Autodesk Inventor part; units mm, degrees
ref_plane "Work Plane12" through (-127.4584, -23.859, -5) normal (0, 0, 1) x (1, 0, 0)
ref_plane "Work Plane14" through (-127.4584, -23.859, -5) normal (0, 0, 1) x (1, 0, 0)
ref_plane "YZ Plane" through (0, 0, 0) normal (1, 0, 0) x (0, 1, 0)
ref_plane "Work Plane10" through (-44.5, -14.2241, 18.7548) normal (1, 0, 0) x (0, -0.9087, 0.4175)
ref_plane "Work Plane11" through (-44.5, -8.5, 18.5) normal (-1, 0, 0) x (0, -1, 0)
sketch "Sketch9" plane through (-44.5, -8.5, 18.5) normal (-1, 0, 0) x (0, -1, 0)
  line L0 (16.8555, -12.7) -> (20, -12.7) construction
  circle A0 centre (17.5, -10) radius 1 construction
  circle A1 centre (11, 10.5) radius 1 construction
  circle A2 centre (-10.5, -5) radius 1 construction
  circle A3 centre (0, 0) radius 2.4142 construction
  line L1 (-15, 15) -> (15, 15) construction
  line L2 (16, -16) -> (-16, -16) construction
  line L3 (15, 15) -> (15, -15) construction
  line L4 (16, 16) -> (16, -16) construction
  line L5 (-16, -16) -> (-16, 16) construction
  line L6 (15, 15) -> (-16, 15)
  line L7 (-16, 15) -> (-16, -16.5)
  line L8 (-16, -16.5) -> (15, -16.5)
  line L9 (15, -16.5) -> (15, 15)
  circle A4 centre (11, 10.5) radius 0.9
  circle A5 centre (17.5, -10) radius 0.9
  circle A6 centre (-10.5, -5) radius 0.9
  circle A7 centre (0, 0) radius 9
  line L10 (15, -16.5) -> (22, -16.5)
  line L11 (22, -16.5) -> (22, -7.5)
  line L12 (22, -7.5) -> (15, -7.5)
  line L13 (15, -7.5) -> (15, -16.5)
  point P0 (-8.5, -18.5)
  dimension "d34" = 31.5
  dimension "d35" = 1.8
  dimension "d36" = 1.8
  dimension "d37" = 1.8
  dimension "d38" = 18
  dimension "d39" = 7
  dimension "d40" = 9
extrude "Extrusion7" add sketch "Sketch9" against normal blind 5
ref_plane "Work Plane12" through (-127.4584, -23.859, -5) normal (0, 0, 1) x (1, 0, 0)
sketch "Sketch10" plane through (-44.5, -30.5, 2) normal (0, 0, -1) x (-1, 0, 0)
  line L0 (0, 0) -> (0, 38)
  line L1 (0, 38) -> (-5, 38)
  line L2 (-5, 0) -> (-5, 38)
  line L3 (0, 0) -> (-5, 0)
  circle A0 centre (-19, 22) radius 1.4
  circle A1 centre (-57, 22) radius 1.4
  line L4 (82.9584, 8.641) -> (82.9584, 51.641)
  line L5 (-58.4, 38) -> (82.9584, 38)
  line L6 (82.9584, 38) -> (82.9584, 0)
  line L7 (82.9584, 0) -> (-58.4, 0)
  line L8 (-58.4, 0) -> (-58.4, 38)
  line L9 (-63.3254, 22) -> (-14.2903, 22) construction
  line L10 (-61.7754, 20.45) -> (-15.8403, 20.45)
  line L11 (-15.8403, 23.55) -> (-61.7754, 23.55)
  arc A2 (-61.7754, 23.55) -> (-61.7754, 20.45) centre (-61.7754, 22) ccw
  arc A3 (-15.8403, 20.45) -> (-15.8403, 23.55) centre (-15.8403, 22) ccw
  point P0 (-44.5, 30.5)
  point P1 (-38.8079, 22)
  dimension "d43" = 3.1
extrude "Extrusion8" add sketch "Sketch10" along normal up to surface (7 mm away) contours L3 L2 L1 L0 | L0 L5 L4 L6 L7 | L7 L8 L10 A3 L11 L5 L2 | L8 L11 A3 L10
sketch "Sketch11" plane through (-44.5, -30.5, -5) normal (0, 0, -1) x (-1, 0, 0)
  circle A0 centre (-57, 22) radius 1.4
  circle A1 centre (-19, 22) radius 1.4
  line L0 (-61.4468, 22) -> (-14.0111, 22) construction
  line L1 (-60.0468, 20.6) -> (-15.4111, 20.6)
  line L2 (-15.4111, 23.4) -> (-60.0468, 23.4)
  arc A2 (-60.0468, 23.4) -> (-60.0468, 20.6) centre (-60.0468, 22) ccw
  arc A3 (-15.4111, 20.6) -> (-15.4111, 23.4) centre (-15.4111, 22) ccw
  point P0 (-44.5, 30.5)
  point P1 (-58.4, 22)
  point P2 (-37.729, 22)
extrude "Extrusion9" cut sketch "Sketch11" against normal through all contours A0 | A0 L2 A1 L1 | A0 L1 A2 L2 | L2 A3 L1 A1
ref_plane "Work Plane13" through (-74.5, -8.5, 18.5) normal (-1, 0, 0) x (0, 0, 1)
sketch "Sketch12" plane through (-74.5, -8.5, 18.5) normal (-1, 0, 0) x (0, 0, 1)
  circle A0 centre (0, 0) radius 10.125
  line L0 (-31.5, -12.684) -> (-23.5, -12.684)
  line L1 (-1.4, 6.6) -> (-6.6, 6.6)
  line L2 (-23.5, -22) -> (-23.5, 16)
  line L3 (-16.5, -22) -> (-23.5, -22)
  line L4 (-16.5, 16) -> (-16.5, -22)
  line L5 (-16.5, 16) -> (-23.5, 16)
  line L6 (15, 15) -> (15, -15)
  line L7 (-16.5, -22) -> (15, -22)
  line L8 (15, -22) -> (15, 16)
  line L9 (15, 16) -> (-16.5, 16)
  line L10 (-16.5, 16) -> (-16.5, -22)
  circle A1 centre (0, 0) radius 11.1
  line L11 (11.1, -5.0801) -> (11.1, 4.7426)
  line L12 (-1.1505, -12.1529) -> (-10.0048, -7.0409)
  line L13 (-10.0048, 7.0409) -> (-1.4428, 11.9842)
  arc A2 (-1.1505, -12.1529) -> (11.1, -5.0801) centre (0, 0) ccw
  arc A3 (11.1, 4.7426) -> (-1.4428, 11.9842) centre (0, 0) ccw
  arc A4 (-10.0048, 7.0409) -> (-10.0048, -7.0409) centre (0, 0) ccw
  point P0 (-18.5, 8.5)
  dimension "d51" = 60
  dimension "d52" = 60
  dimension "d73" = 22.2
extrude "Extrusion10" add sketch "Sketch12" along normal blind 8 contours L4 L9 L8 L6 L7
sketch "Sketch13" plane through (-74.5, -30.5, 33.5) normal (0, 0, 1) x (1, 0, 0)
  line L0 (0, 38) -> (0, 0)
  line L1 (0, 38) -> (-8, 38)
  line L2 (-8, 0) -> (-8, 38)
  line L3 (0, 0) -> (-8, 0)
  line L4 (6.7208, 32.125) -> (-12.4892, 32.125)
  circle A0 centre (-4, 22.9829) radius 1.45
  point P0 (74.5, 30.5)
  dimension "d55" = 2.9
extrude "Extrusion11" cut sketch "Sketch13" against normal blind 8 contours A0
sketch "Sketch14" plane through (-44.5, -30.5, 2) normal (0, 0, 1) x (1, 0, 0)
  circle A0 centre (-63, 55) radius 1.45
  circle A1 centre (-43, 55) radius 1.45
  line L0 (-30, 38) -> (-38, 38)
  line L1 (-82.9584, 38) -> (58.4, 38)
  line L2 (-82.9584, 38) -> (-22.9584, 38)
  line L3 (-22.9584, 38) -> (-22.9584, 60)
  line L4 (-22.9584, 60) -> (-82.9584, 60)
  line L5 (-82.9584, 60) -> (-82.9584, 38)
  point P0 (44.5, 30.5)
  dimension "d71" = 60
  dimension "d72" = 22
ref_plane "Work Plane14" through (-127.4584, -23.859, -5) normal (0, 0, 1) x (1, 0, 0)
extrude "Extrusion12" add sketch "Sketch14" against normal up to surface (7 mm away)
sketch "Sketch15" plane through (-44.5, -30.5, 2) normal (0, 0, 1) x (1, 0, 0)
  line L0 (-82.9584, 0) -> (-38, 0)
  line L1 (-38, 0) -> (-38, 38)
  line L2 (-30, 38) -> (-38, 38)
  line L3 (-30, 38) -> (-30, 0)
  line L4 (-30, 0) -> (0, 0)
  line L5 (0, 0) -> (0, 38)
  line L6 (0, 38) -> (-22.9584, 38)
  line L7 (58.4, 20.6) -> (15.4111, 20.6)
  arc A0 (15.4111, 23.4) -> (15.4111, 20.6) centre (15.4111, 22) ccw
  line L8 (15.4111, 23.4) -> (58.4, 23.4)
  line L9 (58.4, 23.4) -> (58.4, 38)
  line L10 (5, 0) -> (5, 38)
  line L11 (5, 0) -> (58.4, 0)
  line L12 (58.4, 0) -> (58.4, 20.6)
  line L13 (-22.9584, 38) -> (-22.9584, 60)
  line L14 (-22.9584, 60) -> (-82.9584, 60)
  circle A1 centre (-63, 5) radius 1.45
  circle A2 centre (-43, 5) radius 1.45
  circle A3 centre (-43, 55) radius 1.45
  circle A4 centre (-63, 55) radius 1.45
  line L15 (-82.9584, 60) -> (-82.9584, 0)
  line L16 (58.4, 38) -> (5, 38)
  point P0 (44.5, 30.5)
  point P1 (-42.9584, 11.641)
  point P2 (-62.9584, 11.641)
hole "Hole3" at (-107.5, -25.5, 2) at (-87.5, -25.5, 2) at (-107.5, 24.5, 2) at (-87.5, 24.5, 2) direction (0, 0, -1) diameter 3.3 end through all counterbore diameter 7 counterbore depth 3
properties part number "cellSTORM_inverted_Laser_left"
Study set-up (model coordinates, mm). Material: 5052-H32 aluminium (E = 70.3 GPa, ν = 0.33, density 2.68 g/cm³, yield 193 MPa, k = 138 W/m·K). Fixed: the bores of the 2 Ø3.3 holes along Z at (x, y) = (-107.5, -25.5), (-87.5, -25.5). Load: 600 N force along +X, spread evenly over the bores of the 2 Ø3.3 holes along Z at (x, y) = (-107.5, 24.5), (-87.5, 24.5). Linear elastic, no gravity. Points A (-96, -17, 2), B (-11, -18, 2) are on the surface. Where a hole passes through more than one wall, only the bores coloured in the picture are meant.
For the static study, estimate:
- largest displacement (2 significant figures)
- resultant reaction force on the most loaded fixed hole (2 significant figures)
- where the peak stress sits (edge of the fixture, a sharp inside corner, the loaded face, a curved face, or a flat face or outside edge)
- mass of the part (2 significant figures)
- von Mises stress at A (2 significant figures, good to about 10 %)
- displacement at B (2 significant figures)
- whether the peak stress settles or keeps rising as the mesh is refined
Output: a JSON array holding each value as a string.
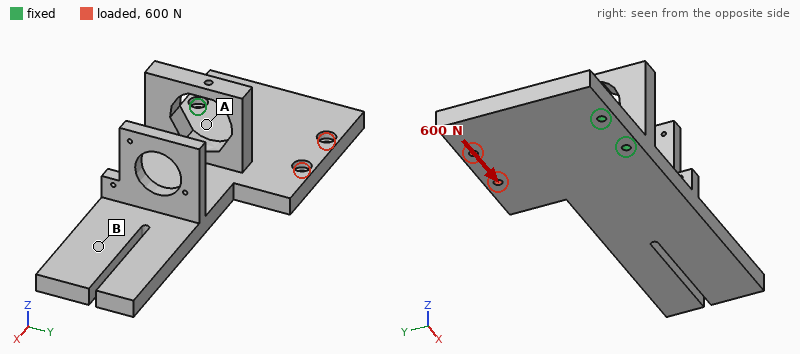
["67 µm", "1.4 kN", "edge of the fixture", "150 g", "6.0 MPa", "48 µm", "keeps rising"]
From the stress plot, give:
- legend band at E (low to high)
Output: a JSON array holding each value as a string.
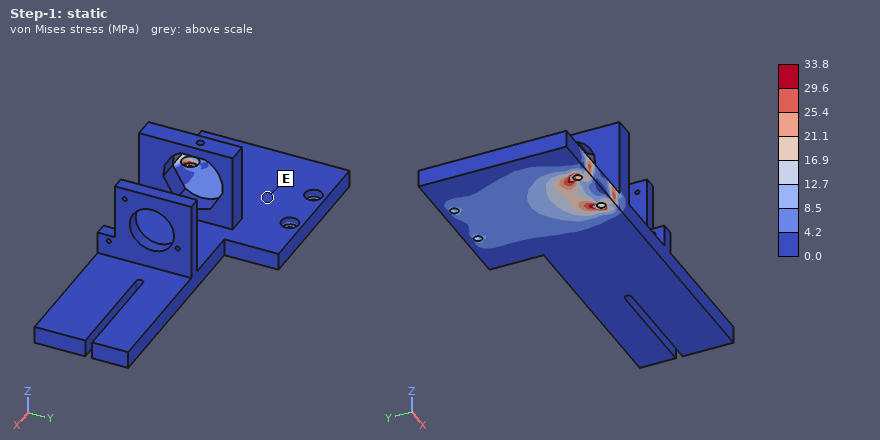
["0.0 to 4.2 MPa"]
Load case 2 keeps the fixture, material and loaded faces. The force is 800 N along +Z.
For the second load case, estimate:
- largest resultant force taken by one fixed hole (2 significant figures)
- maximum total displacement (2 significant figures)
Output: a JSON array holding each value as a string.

["490 N", "0.61 mm"]
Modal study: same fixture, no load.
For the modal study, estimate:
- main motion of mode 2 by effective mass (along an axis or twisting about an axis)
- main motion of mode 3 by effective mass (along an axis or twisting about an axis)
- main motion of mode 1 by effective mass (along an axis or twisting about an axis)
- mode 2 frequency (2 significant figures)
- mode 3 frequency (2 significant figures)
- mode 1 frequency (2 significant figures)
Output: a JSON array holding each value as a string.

["along Z", "along Y", "along Z", "1100 Hz", "1700 Hz", "490 Hz"]
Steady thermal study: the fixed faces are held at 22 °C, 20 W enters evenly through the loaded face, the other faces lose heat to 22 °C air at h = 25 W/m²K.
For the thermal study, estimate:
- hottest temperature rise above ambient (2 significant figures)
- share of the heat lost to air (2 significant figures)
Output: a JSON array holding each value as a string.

["23 K", "20 %"]
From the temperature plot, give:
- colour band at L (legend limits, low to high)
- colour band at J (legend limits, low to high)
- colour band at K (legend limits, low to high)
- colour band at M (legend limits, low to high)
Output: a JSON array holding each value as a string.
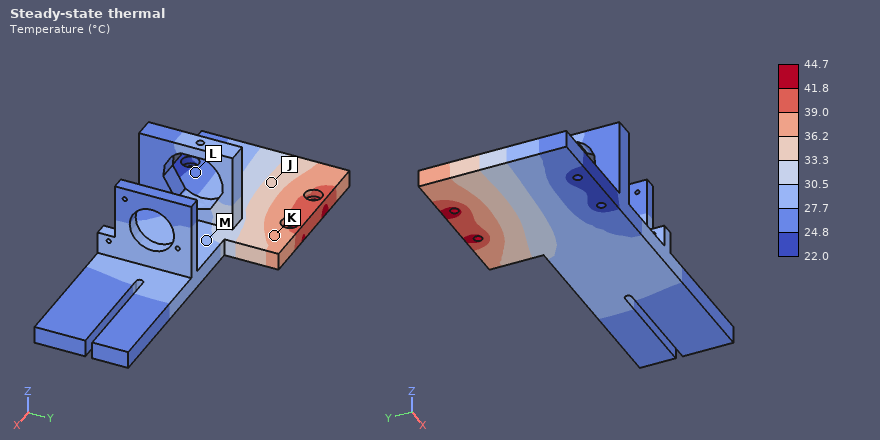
["24.8 to 27.7 °C", "33.3 to 36.2 °C", "36.2 to 39.0 °C", "27.7 to 30.5 °C"]
